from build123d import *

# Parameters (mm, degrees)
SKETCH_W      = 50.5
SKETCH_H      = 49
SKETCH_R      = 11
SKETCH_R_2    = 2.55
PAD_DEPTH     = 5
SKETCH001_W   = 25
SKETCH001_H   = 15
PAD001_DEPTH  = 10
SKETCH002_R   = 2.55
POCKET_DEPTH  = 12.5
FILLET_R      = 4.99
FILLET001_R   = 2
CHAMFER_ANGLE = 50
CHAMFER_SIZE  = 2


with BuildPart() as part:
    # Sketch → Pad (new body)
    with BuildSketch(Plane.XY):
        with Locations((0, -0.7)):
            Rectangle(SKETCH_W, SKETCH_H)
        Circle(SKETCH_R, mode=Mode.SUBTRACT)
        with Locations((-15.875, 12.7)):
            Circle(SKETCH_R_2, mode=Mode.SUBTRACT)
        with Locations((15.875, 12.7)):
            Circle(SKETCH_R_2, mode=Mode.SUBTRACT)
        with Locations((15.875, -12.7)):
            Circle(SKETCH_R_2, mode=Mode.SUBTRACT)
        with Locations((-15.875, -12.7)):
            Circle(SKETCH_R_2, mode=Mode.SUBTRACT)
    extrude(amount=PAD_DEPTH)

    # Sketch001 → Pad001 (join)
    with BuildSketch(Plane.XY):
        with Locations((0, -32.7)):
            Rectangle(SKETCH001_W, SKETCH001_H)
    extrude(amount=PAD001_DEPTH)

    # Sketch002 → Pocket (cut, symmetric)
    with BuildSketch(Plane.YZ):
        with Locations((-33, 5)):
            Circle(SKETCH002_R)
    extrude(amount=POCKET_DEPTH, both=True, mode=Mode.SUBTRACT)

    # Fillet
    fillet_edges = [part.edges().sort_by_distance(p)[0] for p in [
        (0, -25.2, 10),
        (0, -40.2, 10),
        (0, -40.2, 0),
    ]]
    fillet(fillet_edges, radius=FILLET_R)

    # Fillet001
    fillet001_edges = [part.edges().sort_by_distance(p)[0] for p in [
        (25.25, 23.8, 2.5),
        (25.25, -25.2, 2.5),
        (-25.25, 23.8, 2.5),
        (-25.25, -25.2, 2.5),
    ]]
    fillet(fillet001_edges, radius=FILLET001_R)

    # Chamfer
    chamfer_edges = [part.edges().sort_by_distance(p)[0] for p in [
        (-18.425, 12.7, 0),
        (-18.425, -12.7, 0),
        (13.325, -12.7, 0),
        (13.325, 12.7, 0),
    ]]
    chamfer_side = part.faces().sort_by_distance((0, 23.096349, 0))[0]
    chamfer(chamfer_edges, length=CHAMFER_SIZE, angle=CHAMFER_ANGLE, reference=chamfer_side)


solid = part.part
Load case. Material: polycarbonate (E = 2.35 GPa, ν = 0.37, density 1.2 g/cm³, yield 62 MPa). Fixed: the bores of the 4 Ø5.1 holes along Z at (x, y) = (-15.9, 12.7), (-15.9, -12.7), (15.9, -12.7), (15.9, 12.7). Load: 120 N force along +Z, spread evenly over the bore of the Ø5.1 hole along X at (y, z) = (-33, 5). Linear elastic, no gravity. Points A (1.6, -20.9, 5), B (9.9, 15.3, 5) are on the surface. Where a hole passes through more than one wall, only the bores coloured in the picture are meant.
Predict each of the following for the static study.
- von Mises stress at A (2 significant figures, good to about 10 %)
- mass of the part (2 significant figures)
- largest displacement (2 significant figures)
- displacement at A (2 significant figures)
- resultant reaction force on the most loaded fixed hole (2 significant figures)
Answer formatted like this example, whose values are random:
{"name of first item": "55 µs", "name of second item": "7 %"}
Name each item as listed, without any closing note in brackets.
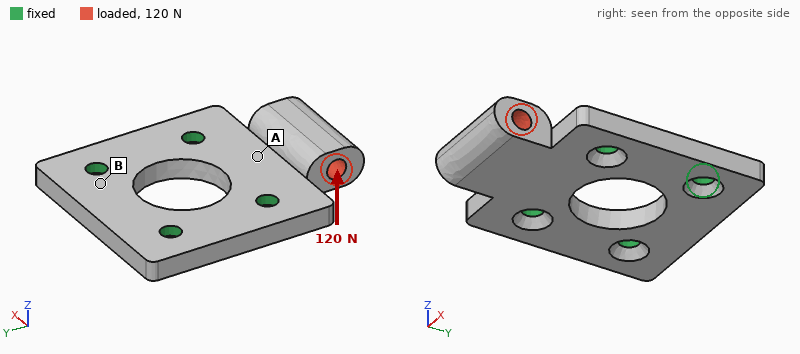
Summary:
{"von Mises stress at A": "7.9 MPa", "mass of the part": "15 g", "largest displacement": "0.86 mm", "displacement at A": "0.19 mm", "resultant reaction force on the most loaded fixed hole": "86 N"}
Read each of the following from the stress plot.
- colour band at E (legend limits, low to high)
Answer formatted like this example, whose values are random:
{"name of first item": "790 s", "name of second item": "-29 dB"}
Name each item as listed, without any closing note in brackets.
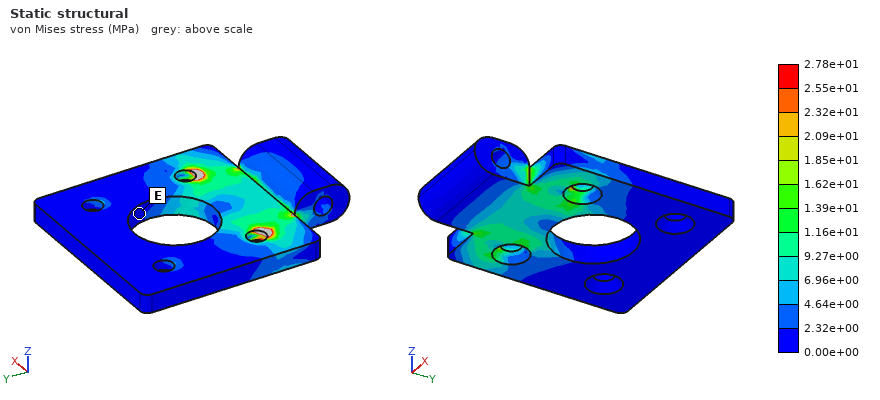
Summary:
{"colour band at E": "0.00e+00 to 2.32e+00 MPa"}
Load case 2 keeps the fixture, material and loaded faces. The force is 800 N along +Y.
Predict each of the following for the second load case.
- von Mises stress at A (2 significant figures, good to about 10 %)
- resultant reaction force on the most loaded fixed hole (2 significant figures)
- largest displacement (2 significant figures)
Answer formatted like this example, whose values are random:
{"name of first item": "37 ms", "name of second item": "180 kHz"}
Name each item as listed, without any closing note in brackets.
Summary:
{"von Mises stress at A": "14 MPa", "resultant reaction force on the most loaded fixed hole": "420 N", "largest displacement": "0.85 mm"}
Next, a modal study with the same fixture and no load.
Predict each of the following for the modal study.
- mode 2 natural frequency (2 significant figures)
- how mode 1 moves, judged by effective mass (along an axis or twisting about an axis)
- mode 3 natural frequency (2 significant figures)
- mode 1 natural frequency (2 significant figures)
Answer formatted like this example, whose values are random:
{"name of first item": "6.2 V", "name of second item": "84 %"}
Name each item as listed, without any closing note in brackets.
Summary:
{"mode 2 natural frequency": "3900 Hz", "how mode 1 moves, judged by effective mass": "along Z", "mode 3 natural frequency": "4700 Hz", "mode 1 natural frequency": "1200 Hz"}
